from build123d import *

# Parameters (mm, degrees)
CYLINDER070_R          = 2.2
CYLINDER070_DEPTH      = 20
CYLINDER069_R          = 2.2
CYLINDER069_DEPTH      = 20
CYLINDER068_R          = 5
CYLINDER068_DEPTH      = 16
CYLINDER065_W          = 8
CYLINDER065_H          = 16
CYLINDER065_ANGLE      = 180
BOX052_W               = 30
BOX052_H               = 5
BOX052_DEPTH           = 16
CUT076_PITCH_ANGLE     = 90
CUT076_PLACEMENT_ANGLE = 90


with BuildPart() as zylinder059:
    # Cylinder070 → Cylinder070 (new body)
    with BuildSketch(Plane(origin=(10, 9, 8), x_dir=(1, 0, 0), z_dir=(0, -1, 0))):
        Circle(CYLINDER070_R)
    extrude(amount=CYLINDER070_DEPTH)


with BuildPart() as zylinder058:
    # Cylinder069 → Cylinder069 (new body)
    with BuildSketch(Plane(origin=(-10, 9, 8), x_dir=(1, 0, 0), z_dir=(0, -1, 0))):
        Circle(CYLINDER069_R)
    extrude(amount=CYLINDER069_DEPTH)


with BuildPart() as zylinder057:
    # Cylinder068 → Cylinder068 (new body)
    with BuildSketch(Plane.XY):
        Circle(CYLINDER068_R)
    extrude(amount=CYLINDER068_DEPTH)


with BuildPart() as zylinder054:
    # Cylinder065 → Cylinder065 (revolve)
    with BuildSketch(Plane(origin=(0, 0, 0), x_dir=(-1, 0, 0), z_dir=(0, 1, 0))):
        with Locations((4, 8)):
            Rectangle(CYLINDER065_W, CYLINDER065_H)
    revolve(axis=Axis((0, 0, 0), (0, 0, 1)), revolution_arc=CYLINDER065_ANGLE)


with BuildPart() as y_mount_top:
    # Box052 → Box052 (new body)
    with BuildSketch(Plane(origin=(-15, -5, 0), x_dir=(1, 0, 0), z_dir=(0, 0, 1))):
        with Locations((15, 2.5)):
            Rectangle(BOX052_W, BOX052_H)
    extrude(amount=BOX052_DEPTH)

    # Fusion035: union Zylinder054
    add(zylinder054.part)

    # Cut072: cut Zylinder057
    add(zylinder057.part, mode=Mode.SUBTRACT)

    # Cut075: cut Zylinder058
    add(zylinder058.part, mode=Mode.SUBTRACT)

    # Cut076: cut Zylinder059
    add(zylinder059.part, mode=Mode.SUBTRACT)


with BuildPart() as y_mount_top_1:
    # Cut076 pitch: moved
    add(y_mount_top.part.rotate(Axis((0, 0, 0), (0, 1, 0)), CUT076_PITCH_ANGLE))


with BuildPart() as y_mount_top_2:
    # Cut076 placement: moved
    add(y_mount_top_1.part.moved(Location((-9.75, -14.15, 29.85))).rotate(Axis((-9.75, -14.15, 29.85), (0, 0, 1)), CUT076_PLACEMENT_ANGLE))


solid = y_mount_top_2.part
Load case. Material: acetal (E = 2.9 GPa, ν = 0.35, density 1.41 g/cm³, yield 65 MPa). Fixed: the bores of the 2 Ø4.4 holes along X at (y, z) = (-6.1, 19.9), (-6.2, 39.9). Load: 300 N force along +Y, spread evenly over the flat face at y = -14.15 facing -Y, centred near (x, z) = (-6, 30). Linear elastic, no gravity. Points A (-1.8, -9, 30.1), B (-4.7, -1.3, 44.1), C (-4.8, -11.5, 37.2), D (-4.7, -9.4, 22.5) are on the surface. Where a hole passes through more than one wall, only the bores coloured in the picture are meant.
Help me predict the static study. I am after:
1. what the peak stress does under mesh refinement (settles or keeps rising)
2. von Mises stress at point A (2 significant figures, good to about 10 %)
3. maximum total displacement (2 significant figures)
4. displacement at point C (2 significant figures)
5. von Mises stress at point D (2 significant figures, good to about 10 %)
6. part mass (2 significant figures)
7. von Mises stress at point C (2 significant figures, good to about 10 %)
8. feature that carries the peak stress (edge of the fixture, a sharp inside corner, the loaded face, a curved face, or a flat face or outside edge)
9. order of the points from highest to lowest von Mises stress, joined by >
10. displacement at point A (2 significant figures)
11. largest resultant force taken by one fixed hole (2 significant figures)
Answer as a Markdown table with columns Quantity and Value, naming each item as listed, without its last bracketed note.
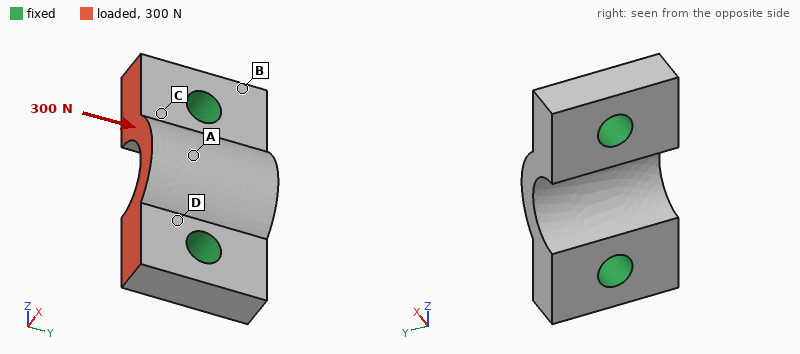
| Quantity | Value |
|---|---|
| what the peak stress does under mesh refinement | keeps rising |
| von Mises stress at point A | 1.8 MPa |
| maximum total displacement | 26 µm |
| displacement at point C | 8.3 µm |
| von Mises stress at point D | 4.5 MPa |
| part mass | 2.9 g |
| von Mises stress at point C | 3.4 MPa |
| feature that carries the peak stress | edge of the fixture |
| order of the points from highest to lowest von Mises stress, joined by > | D > C > A > B |
| displacement at point A | 18 µm |
| largest resultant force taken by one fixed hole | 150 N |
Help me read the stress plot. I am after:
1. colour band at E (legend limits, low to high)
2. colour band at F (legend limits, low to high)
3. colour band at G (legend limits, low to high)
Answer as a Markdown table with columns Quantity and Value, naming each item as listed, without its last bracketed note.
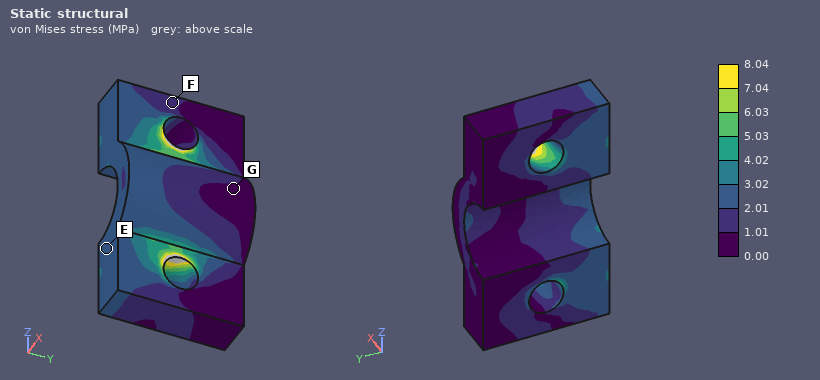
| Quantity | Value |
|---|---|
| colour band at E | 2.01 to 3.02 MPa |
| colour band at F | 1.01 to 2.01 MPa |
| colour band at G | 0.00 to 1.01 MPa |
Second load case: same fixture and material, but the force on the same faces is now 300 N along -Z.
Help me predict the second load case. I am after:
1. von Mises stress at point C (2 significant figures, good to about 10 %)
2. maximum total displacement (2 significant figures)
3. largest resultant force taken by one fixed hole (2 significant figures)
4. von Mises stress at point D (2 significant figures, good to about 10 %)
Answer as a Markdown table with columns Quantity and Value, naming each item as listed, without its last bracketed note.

| Quantity | Value |
|---|---|
| von Mises stress at point C | 7.8 MPa |
| maximum total displacement | 39 µm |
| largest resultant force taken by one fixed hole | 160 N |
| von Mises stress at point D | 7.6 MPa |
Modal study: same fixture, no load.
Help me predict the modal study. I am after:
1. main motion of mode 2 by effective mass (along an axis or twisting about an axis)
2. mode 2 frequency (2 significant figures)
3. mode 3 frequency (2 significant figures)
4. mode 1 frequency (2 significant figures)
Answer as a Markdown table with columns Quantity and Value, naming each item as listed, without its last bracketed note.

| Quantity | Value |
|---|---|
| main motion of mode 2 by effective mass | along X |
| mode 2 frequency | 16 kHz |
| mode 3 frequency | 17 kHz |
| mode 1 frequency | 11 kHz |
